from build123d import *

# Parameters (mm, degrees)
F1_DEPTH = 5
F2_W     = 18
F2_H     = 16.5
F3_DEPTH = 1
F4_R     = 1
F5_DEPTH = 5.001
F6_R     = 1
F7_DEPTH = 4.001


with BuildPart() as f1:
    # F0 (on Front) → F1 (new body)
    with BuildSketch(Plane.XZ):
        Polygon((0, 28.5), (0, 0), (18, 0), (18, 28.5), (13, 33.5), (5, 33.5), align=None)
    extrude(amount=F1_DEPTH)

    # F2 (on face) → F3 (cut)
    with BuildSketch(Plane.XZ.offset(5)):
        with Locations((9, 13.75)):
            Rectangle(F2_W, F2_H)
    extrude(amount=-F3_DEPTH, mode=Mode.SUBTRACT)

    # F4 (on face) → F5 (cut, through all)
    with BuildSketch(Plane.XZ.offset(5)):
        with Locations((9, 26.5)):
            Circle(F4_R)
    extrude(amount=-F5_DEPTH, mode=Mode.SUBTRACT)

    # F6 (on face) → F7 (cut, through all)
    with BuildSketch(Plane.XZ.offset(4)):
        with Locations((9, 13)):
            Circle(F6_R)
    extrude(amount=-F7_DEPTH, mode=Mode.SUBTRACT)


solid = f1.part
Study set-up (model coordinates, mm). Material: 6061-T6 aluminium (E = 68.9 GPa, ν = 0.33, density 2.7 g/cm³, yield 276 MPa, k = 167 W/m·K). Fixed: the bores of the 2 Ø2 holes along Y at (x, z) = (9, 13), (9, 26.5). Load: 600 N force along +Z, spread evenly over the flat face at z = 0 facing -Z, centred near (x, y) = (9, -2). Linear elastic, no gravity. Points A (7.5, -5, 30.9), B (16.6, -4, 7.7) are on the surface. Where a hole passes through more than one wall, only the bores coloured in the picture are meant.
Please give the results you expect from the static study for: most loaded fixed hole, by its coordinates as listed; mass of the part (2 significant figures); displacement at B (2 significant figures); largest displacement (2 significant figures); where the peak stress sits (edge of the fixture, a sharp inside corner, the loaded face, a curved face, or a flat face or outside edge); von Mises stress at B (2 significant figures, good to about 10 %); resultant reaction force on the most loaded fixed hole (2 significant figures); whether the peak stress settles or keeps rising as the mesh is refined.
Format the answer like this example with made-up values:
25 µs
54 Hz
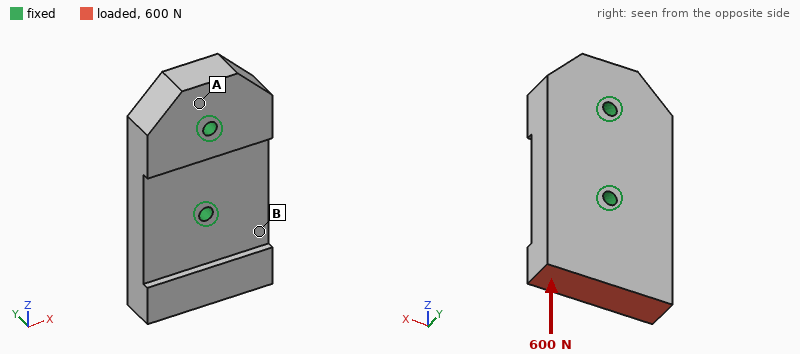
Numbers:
(9, 13)
6.9 g
2.2 µm
5.3 µm
edge of the fixture
12 MPa
440 N
keeps rising
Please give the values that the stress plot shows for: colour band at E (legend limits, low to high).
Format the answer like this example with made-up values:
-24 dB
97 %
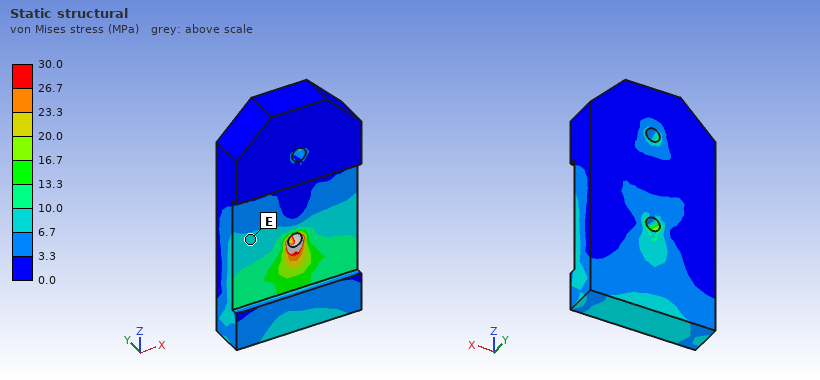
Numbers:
6.7 to 10.0 MPa
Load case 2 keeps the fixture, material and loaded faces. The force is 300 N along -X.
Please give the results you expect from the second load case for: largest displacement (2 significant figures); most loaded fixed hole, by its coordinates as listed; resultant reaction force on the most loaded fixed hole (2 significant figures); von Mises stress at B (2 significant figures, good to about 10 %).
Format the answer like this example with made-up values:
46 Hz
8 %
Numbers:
10 µm
(9, 13)
550 N
12 MPa
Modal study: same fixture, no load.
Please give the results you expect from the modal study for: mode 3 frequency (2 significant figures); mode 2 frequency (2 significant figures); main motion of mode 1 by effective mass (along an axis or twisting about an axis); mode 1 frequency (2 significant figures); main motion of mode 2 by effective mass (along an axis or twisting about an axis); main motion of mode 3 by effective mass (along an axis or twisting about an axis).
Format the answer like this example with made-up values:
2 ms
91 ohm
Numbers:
26 kHz
19 kHz
along Y
14 kHz
twisting about Z
along X
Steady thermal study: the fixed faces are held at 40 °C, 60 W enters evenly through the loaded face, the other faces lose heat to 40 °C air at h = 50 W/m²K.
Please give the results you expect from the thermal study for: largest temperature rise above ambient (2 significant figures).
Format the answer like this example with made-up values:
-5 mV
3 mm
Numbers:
71 K
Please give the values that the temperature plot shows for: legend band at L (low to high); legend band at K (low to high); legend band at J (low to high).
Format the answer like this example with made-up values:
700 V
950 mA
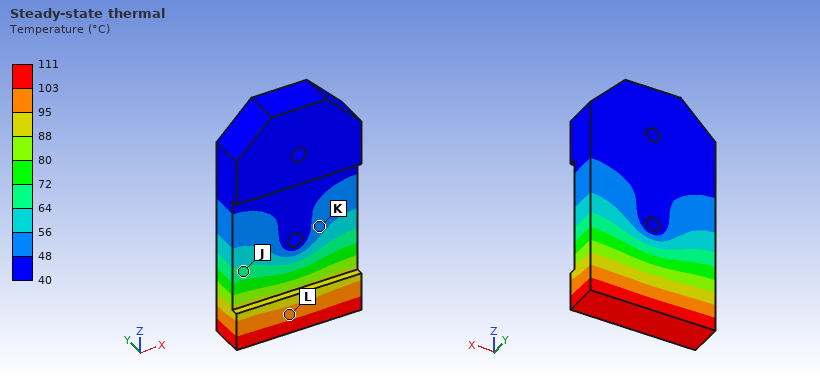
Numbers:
95 to 103 °C
48 to 56 °C
64 to 72 °C
